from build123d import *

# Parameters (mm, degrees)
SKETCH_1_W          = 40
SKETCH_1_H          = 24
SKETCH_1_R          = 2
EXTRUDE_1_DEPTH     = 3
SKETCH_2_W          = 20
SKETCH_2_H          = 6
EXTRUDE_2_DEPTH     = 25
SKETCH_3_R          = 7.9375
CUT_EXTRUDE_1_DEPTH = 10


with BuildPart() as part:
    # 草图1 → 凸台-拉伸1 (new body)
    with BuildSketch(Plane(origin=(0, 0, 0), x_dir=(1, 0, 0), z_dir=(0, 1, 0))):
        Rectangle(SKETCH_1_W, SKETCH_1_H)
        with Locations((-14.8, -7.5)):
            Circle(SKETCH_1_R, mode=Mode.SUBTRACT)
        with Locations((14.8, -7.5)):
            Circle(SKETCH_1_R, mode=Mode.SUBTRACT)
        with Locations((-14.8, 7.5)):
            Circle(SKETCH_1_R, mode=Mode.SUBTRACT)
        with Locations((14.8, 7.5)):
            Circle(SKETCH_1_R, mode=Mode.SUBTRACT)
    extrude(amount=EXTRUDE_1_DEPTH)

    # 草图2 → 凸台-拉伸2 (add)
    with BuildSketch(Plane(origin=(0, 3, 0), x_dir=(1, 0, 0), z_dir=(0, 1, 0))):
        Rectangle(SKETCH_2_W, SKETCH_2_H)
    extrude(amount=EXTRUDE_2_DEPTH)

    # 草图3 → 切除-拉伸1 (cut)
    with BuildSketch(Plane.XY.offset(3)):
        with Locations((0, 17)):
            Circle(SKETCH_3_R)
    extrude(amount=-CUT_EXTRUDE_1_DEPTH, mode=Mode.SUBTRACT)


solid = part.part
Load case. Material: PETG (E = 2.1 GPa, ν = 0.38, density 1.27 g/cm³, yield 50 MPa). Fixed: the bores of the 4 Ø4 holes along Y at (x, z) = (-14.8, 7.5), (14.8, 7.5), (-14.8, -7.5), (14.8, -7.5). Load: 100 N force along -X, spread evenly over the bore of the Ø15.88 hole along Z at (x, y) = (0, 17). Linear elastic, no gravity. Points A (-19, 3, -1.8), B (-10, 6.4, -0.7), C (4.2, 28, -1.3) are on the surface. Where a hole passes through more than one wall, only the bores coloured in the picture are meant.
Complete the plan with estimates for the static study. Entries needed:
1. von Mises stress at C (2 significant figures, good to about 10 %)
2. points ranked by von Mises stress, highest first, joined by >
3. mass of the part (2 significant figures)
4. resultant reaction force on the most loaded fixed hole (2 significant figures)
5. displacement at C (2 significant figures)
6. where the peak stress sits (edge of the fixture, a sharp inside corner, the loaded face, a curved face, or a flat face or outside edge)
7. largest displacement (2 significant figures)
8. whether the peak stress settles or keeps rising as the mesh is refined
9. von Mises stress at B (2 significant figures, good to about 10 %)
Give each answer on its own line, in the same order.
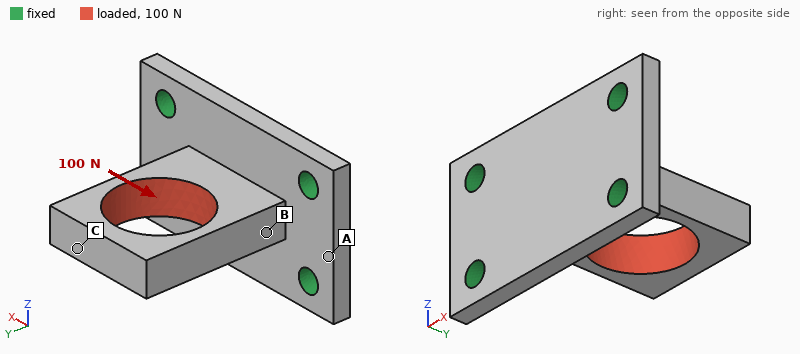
3.7 MPa
B > C > A
5.8 g
43 N
0.36 mm
edge of the fixture
0.37 mm
keeps rising
6.4 MPa
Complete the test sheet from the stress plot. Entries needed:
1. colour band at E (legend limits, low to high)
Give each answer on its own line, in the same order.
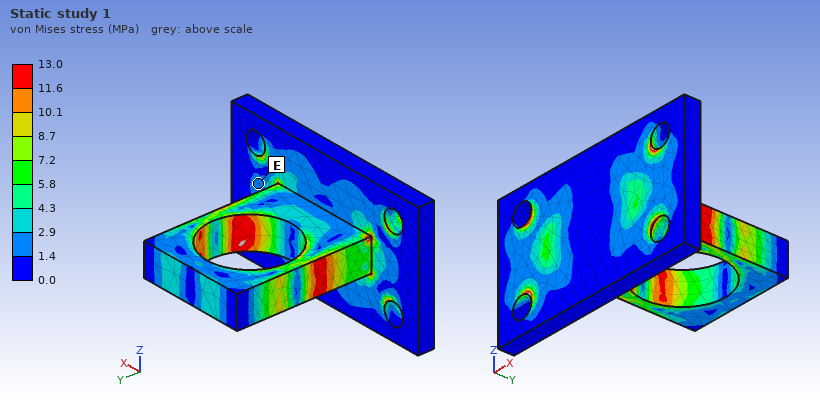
1.4 to 2.9 MPa
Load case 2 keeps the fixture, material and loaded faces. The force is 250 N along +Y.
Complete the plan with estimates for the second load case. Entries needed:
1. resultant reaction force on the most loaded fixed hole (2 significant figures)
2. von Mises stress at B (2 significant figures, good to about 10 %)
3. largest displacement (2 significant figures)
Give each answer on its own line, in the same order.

65 N
7.4 MPa
0.19 mm
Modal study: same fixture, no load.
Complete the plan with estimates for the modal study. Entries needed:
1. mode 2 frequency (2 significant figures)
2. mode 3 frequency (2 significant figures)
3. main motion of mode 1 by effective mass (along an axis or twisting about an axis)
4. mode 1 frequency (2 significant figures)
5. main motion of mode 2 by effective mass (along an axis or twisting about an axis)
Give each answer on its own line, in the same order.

2100 Hz
2900 Hz
along Z
1300 Hz
along X
